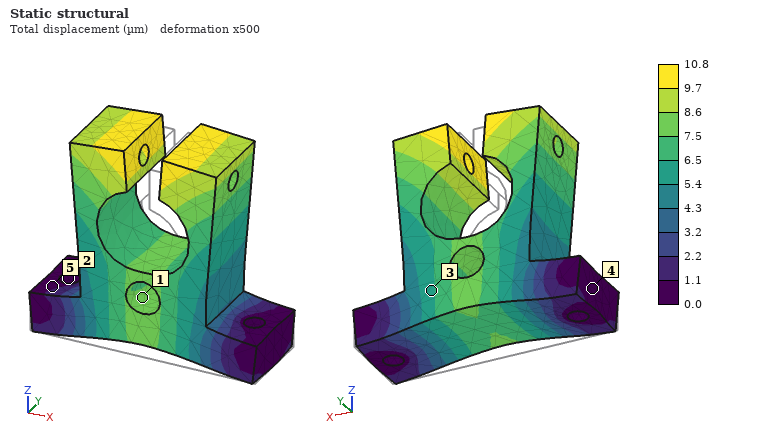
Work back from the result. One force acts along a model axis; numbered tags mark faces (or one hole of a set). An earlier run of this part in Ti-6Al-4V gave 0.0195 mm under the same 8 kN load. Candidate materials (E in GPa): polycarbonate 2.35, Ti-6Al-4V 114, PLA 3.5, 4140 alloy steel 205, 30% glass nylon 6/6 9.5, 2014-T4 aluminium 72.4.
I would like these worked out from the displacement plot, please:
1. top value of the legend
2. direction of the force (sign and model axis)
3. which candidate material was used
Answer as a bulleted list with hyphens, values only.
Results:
- 10.8 µm
- +Z
- 4140 alloy steel
